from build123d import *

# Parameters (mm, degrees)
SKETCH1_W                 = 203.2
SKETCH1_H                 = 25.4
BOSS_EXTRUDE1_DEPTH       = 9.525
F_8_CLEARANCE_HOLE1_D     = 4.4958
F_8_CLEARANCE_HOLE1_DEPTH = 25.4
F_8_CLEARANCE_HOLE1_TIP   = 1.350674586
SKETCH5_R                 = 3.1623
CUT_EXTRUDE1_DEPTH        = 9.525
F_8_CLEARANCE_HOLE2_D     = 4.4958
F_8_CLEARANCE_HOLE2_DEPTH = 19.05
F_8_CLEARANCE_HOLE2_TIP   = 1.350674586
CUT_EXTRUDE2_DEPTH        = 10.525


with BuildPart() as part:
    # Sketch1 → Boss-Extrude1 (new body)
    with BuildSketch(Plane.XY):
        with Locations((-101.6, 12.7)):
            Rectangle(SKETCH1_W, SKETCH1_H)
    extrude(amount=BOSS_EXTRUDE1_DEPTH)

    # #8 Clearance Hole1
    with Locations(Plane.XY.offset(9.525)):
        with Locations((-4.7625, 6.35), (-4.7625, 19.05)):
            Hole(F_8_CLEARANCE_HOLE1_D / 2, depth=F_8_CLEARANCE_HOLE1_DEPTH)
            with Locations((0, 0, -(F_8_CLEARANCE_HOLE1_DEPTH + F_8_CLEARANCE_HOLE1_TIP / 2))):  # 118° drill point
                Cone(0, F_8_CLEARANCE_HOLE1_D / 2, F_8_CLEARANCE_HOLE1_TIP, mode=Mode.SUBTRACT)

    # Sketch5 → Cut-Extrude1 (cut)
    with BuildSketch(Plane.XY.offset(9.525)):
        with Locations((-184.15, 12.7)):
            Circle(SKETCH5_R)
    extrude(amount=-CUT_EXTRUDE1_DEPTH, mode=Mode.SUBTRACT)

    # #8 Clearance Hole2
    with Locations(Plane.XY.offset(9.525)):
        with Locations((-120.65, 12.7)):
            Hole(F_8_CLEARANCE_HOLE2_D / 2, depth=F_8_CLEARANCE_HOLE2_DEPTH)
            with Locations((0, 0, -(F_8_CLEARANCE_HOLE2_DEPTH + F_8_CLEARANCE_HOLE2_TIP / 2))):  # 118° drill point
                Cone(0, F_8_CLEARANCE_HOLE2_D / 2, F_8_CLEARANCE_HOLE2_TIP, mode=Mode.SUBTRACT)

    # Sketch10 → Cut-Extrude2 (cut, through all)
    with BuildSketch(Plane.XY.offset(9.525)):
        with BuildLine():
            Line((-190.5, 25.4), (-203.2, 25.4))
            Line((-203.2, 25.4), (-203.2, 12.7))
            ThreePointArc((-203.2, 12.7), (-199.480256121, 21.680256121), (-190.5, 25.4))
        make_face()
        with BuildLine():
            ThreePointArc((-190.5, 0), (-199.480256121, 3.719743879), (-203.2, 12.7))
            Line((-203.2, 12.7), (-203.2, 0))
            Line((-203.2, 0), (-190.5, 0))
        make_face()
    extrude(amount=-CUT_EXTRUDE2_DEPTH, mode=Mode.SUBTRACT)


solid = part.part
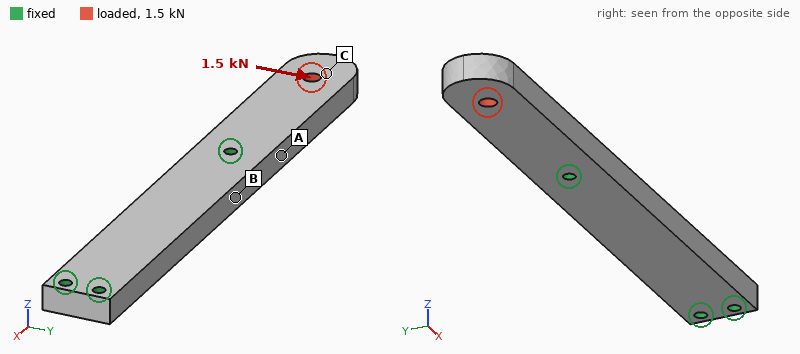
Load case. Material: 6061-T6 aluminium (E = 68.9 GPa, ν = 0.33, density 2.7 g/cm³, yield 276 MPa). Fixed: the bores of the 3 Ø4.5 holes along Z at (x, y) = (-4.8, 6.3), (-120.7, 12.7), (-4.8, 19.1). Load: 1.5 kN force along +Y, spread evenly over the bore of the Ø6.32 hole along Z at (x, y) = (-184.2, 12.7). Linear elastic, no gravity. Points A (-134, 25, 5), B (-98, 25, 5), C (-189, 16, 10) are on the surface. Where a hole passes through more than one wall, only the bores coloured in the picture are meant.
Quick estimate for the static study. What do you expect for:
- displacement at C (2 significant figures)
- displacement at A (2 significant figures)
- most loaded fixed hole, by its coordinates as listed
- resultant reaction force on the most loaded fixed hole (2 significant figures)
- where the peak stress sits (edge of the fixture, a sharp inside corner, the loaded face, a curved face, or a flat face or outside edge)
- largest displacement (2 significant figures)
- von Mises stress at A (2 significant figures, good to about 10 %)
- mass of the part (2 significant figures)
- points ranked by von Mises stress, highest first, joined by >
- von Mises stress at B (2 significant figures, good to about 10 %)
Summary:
0.33 mm
0.061 mm
(-120.7, 12.7)
2.2 kN
edge of the fixture
0.40 mm
75 MPa
130 g
A > B > C
42 MPa
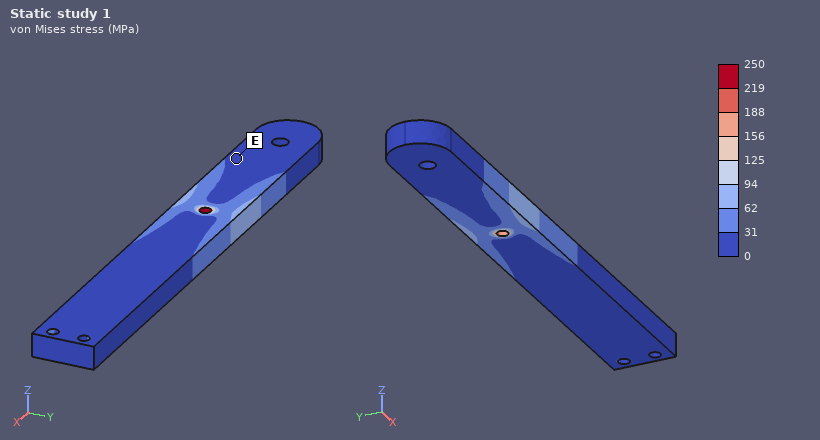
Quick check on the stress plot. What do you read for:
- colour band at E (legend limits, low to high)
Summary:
0 to 31 MPa
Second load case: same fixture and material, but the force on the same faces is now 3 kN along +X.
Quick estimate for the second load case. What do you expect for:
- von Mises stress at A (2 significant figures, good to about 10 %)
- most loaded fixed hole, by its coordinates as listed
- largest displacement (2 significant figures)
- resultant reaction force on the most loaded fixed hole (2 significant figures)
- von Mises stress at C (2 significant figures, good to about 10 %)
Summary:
10 MPa
(-120.7, 12.7)
14 µm
2.8 kN
11 MPa
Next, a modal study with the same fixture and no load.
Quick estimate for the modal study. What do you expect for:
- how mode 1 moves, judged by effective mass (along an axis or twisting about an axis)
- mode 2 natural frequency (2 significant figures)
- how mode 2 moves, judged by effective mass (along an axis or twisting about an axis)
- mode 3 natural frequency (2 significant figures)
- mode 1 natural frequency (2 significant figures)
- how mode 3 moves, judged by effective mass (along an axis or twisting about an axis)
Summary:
along Z
2200 Hz
along Y
3500 Hz
1200 Hz
along Z
